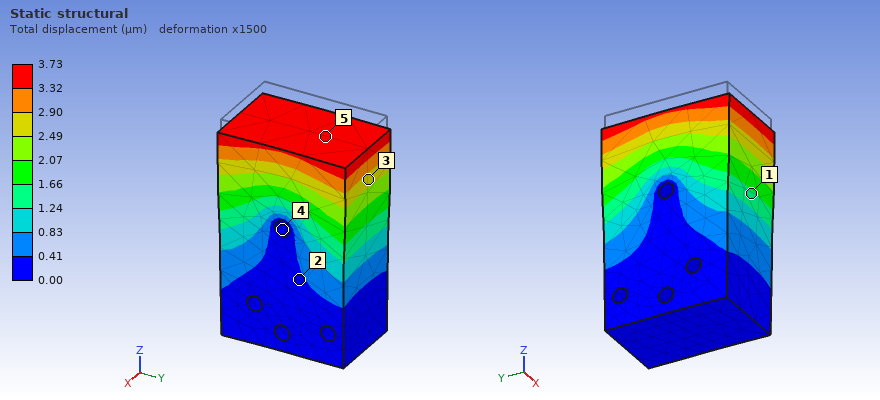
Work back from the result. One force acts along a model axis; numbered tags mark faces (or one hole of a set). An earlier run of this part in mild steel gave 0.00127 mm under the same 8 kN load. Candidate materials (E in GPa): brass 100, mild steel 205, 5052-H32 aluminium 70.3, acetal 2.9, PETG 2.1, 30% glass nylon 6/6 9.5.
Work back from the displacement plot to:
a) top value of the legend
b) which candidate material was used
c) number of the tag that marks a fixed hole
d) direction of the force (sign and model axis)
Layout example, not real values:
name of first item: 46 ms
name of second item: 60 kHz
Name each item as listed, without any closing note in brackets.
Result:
top value of the legend: 3.73 µm
which candidate material was used: 5052-H32 aluminium
number of the tag that marks a fixed hole: 4
direction of the force: -Z
